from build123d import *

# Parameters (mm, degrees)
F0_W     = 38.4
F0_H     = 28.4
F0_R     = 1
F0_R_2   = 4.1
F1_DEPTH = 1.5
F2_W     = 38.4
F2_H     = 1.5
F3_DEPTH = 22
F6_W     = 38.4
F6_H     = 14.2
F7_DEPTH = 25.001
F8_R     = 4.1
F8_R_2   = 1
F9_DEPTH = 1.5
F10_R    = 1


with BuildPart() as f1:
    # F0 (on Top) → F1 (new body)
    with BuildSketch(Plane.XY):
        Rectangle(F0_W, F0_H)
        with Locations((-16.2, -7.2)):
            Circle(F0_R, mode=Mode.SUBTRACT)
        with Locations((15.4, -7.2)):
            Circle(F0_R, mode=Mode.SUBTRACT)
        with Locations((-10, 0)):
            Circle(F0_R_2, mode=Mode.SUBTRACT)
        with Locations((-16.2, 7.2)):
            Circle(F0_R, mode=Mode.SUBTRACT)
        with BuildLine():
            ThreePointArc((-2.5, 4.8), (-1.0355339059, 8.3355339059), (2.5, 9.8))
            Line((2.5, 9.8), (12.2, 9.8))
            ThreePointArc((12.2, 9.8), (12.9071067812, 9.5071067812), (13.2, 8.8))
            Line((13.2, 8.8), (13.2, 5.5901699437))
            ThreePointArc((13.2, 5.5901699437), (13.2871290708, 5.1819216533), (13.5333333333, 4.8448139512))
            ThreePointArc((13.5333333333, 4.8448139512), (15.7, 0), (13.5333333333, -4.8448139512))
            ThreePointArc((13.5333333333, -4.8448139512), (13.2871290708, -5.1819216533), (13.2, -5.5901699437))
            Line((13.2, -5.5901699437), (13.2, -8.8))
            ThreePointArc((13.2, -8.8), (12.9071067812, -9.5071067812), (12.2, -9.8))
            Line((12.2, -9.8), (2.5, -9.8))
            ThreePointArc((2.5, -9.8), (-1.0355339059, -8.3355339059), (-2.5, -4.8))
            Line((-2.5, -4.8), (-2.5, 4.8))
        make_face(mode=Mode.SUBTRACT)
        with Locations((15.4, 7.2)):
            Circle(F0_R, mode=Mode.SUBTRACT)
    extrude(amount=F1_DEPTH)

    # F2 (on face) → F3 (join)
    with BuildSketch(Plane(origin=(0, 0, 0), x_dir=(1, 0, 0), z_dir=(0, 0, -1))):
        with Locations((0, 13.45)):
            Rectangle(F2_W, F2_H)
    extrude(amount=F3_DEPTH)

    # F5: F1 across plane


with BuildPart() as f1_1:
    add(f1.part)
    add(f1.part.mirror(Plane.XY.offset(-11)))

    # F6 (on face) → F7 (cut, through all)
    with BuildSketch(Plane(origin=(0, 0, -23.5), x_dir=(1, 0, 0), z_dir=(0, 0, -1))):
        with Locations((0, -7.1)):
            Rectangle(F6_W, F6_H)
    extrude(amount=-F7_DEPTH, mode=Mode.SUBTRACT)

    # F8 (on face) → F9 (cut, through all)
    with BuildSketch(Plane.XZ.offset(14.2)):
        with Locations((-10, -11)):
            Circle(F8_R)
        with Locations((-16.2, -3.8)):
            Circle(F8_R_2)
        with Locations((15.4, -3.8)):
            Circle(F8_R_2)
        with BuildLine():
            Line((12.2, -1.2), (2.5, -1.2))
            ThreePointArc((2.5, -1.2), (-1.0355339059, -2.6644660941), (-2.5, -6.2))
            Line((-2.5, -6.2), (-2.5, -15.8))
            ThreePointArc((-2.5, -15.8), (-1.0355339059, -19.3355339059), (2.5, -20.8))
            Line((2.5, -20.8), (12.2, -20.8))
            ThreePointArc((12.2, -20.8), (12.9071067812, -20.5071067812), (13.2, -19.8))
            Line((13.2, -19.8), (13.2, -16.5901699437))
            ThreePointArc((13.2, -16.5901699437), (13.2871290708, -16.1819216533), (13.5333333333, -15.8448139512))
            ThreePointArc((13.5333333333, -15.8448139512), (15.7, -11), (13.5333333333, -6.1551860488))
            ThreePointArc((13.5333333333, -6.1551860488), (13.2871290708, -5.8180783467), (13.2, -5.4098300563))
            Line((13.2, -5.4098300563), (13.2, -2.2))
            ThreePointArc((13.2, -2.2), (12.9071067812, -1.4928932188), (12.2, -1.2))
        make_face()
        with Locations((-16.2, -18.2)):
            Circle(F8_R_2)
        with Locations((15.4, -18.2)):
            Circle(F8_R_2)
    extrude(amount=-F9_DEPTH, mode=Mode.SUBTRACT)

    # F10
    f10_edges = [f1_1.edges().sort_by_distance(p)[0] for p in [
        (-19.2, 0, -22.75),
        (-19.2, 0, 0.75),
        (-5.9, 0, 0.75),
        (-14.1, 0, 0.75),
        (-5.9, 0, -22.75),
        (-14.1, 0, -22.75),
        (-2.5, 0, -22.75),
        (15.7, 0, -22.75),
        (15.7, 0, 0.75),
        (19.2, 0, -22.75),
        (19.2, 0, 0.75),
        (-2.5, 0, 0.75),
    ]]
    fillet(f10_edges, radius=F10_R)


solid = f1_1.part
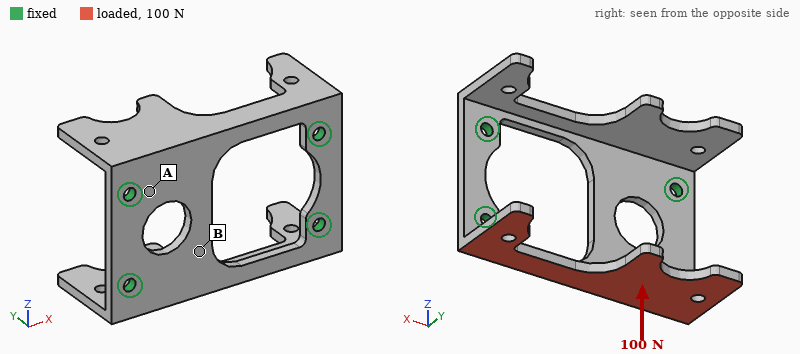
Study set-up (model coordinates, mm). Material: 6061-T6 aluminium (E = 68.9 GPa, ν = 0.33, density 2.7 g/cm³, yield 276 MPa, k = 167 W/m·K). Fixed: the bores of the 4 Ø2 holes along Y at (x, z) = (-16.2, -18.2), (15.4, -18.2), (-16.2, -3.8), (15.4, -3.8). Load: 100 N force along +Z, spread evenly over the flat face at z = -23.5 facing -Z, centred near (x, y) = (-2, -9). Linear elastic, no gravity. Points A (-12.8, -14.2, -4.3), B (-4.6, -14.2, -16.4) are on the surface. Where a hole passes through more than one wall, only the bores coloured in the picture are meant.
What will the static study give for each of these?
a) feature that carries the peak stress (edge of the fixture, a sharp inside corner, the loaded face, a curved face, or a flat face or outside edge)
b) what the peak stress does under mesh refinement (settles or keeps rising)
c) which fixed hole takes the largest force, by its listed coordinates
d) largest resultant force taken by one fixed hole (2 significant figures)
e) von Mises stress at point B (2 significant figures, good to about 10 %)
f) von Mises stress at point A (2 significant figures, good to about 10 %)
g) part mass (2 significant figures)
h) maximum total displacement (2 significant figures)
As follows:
edge of the fixture
keeps rising
(-16.2, -18.2)
50 N
24 MPa
9.7 MPa
4.8 g
0.11 mm
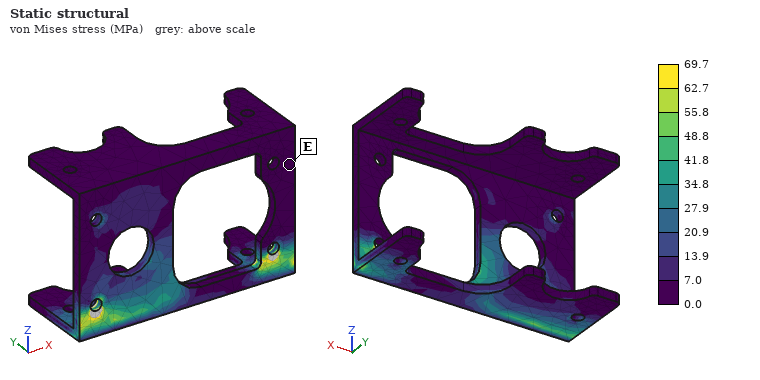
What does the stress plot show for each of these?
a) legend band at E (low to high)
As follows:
0.0 to 7.0 MPa
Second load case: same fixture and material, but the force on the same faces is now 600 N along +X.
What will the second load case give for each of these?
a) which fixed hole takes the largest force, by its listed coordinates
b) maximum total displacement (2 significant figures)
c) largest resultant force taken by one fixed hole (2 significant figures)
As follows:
(-16.2, -18.2)
63 µm
430 N
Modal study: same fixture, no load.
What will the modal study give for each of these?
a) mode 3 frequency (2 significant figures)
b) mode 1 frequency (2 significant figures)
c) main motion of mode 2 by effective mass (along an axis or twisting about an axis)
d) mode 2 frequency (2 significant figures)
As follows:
6300 Hz
5100 Hz
along Z
5300 Hz
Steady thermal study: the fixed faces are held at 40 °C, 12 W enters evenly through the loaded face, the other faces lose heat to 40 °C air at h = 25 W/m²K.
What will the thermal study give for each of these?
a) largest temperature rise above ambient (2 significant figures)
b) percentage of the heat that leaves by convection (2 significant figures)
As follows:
25 K
3.3 %
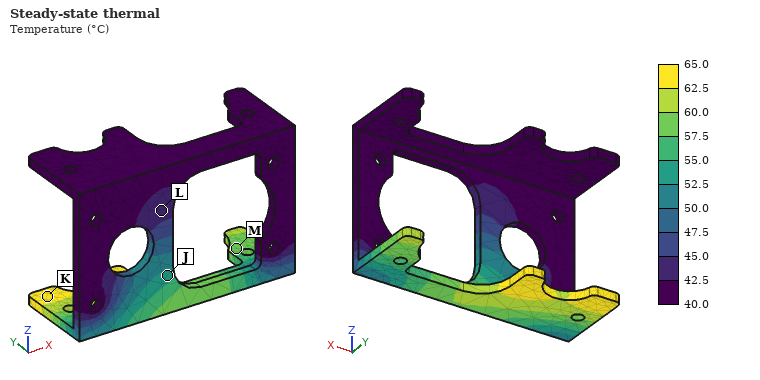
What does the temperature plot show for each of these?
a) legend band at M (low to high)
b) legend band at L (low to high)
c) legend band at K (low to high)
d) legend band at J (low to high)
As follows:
57.5 to 60.0 °C
42.5 to 45.0 °C
62.5 to 65.0 °C
52.5 to 55.0 °C
